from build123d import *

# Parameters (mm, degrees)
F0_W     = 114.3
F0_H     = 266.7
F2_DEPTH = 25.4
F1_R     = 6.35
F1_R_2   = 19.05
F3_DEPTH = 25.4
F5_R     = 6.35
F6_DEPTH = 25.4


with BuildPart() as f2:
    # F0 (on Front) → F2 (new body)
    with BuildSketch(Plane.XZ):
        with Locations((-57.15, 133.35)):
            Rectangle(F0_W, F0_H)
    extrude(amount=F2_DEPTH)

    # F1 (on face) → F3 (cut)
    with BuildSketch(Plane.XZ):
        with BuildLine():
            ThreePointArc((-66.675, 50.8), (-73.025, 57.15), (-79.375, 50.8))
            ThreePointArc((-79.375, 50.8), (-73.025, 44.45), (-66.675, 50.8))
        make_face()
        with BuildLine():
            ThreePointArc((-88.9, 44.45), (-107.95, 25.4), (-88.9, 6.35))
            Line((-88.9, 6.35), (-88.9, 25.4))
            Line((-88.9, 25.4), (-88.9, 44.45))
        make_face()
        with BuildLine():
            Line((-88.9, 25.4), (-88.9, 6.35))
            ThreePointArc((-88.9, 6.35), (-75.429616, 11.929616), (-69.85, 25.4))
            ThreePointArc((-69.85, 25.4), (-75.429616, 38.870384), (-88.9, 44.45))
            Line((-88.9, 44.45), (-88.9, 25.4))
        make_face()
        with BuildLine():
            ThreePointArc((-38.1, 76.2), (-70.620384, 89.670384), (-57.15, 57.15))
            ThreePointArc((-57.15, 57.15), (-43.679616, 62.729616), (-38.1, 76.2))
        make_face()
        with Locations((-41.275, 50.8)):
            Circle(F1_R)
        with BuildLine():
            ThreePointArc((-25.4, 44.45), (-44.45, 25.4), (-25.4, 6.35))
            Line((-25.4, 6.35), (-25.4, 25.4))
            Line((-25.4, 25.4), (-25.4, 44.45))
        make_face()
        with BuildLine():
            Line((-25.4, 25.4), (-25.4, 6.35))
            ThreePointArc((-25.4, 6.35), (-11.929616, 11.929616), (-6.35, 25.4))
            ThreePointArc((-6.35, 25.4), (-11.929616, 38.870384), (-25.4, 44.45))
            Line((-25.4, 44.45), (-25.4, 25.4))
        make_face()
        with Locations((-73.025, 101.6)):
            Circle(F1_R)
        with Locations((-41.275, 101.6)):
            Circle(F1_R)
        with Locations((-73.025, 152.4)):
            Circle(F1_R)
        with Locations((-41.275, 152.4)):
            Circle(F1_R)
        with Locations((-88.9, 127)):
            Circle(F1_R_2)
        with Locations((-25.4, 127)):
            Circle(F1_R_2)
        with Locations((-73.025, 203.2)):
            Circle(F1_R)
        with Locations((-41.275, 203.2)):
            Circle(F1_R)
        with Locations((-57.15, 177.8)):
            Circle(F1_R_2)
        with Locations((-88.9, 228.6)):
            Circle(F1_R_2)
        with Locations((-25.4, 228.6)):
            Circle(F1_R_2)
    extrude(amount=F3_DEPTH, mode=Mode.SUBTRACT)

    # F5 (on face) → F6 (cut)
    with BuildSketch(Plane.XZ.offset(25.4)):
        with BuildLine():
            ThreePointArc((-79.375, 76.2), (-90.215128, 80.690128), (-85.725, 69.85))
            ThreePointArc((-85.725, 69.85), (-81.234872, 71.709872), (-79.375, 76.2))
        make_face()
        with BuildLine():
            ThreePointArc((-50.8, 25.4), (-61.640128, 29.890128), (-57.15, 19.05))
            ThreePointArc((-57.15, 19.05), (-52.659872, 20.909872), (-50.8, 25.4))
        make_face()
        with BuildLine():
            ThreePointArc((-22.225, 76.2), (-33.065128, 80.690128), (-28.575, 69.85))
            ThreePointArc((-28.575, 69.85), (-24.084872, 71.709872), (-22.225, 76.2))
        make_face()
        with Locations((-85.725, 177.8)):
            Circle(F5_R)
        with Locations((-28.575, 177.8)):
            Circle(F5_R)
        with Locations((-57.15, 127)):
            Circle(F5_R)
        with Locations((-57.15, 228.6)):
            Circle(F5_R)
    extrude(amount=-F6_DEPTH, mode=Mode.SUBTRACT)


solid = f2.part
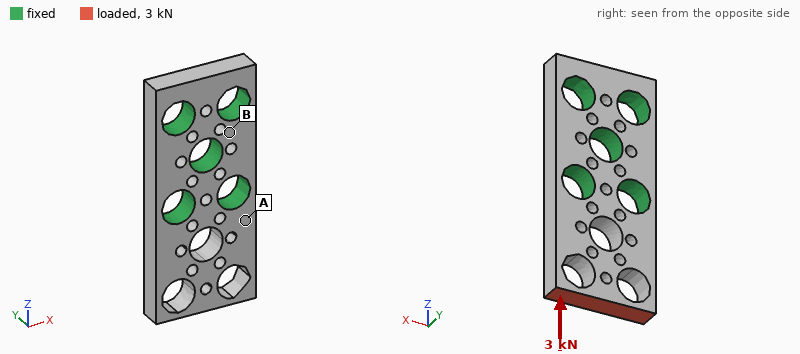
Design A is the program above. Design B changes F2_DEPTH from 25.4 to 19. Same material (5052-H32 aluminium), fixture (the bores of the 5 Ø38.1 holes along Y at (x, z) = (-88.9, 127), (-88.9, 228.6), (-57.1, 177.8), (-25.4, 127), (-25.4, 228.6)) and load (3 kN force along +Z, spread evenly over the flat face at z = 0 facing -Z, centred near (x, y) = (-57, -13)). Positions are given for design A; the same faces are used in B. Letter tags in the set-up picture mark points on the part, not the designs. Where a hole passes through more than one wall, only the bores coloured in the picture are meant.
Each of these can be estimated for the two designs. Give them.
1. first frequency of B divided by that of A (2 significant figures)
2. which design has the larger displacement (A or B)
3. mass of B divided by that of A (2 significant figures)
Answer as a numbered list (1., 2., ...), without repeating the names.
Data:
1. 0.78
2. B
3. 0.75
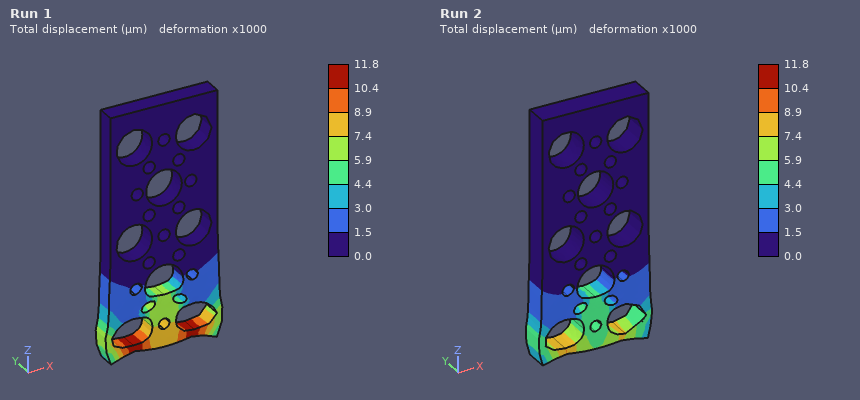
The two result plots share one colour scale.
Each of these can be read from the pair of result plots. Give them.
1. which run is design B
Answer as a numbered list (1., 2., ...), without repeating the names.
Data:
1. Run 1
